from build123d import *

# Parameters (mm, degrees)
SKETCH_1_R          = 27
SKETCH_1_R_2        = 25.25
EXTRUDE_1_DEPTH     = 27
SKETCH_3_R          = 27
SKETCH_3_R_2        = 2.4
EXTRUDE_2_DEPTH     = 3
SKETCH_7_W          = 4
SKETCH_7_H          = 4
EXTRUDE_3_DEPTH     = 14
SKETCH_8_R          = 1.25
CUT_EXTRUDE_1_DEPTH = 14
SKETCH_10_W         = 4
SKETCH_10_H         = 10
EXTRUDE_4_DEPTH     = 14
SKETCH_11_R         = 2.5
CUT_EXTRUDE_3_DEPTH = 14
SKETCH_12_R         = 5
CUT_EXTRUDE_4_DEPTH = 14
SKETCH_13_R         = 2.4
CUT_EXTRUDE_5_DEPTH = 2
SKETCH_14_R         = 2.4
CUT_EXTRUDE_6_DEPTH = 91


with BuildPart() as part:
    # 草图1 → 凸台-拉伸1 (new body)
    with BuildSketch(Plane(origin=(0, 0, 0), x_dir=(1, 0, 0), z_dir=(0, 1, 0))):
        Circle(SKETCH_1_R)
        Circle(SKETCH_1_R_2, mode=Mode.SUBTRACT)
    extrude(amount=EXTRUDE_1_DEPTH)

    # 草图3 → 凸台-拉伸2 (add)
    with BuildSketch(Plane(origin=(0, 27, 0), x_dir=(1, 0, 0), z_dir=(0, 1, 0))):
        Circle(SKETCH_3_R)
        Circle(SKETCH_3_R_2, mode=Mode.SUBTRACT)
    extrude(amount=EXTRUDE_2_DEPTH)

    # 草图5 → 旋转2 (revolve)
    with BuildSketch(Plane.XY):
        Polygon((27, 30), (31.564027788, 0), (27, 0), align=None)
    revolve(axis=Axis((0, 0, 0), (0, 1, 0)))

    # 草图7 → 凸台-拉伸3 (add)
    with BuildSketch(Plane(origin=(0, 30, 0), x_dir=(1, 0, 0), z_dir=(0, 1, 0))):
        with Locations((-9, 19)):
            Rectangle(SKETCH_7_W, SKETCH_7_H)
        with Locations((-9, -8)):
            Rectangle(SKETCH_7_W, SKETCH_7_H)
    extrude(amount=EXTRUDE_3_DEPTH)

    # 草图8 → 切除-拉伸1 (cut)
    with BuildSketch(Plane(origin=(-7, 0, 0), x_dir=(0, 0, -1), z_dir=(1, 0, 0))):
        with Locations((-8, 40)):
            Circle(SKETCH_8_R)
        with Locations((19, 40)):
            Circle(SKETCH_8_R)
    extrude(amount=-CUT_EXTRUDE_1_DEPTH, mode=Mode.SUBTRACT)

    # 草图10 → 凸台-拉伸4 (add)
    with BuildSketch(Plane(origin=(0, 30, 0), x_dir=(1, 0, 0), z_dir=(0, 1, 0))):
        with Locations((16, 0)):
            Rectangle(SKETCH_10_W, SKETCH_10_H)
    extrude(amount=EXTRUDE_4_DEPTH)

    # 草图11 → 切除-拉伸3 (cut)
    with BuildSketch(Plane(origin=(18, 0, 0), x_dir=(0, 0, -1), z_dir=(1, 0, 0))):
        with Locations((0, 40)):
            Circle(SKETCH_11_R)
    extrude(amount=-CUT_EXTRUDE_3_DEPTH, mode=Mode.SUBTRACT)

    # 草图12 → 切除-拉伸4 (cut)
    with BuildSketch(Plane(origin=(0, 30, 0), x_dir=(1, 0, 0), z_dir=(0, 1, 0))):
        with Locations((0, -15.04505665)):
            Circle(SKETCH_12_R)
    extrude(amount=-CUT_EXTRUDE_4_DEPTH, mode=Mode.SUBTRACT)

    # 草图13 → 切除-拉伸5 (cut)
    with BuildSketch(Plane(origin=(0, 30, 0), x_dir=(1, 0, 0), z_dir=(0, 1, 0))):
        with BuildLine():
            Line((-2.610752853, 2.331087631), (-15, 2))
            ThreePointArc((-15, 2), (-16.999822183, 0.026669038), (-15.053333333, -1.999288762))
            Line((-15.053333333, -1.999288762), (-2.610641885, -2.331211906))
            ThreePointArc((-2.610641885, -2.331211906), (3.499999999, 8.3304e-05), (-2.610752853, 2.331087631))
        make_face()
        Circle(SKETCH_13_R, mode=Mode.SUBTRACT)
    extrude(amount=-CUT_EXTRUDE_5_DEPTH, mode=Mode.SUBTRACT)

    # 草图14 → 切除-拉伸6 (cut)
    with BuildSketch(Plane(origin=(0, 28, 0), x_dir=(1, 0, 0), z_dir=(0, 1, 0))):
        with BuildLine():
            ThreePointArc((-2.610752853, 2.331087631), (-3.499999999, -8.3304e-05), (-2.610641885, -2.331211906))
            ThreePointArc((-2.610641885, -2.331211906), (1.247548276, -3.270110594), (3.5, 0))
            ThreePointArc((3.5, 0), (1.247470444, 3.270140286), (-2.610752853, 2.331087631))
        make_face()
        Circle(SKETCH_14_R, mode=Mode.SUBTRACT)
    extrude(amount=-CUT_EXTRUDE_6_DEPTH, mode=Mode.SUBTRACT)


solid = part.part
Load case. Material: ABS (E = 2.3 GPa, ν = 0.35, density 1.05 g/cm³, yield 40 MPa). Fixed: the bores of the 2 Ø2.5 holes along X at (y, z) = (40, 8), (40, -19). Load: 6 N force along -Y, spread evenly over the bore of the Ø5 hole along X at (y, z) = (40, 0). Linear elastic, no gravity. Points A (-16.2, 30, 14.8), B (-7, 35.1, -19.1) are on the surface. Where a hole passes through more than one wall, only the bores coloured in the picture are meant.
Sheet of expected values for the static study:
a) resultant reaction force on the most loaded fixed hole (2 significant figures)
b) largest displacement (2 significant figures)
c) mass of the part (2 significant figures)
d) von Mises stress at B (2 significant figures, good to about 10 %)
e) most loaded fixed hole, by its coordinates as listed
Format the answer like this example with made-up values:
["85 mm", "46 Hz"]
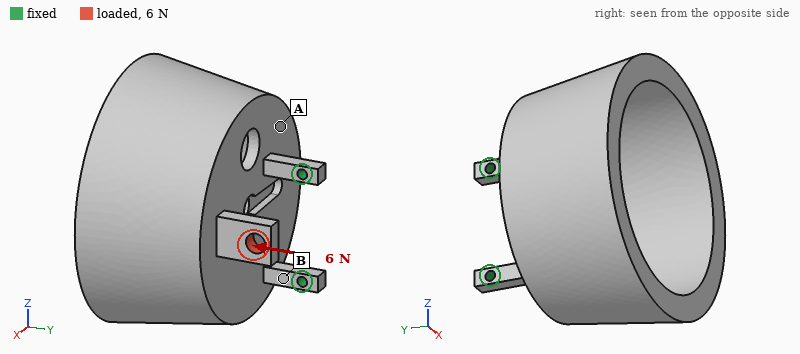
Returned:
["4.2 N", "0.91 mm", "29 g", "7.5 MPa", "(40, 8)"]
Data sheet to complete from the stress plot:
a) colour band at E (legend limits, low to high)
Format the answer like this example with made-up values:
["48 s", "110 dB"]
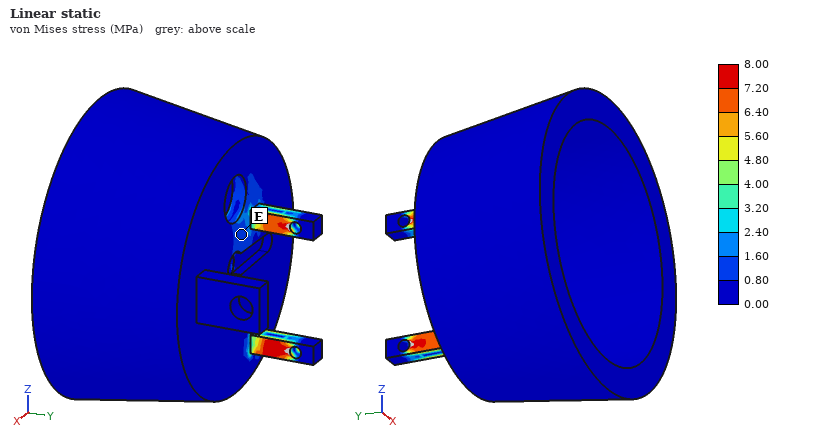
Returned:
["0.80 to 1.60 MPa"]
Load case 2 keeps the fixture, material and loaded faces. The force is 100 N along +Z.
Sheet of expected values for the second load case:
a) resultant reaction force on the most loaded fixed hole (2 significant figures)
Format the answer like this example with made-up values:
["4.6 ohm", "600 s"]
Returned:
["100 N"]
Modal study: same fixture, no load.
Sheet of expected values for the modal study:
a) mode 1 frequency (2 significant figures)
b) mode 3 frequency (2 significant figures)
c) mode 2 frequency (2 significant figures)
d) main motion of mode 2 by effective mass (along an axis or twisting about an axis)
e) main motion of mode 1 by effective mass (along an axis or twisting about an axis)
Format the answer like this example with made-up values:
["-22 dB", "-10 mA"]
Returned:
["96 Hz", "490 Hz", "330 Hz", "along Z", "along X"]
